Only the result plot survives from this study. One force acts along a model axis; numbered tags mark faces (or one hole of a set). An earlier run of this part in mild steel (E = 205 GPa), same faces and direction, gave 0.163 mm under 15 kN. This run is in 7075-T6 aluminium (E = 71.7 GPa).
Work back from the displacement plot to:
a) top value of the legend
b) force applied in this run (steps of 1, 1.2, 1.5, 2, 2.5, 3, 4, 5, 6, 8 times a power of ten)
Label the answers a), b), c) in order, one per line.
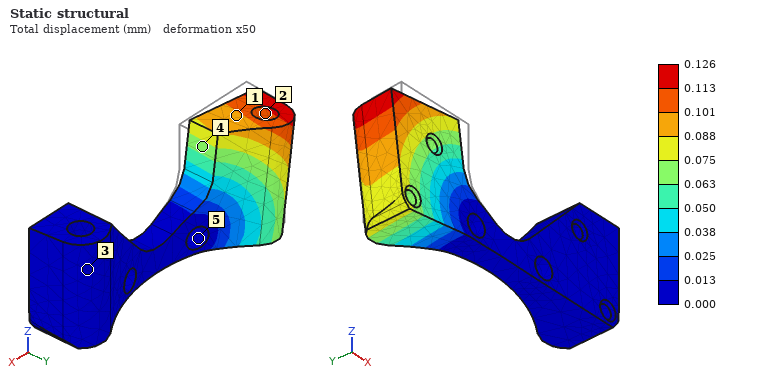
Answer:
a) 0.126 mm
b) 4 kN
